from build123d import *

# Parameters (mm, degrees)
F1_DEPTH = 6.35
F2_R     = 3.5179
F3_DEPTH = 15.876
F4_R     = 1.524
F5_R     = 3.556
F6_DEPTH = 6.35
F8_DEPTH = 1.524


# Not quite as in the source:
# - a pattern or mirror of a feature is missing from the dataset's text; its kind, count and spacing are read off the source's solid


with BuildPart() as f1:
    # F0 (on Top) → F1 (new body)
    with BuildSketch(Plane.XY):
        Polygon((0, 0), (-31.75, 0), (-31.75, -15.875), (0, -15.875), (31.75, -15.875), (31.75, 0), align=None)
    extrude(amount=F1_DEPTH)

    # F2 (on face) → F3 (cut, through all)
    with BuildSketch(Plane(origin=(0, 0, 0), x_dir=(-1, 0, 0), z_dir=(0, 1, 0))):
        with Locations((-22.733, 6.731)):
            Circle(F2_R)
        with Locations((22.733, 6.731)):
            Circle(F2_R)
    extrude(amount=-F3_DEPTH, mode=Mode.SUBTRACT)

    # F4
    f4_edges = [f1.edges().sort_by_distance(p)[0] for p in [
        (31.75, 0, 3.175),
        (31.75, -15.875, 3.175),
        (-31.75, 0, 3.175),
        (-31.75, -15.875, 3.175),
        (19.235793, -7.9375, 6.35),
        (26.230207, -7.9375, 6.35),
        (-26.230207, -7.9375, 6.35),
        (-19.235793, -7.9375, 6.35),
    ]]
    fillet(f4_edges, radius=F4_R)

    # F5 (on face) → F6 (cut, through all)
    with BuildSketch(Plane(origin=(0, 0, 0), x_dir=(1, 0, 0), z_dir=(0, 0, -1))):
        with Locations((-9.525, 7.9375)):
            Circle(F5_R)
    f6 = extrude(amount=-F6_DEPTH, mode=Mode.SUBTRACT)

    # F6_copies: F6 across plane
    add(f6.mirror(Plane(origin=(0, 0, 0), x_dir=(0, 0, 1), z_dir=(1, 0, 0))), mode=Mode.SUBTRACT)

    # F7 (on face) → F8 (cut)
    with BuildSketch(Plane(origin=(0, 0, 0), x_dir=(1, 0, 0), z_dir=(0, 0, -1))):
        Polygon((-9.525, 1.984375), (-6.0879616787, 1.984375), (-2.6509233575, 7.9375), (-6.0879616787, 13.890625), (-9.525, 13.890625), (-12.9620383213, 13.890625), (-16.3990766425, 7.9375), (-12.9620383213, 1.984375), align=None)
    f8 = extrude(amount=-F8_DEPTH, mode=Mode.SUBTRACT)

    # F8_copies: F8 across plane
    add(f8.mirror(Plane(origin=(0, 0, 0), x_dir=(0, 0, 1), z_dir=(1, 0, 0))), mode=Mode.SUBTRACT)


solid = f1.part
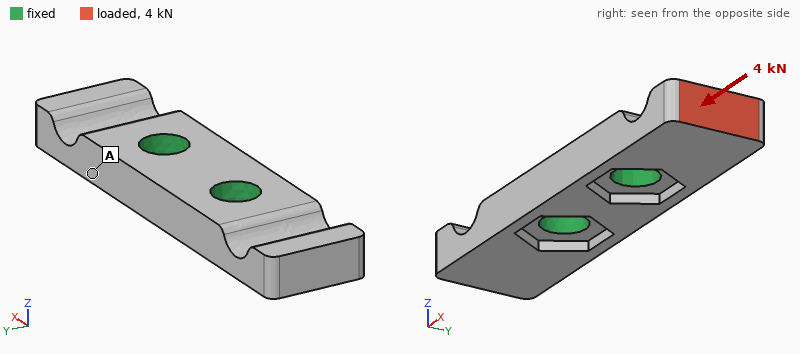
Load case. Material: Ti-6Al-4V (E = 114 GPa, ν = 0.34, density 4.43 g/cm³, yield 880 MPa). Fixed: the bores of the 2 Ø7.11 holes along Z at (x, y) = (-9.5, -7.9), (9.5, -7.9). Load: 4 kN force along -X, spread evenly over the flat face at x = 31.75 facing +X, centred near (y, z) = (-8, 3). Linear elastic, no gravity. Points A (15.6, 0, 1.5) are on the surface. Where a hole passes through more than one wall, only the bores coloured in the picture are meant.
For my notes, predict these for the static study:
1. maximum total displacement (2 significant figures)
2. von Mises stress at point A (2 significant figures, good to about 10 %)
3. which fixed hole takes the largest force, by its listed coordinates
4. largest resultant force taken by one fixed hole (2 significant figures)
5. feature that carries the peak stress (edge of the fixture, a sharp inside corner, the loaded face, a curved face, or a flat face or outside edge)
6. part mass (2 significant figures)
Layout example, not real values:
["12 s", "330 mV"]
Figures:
["59 µm", "42 MPa", "(9.5, -7.9)", "3.7 kN", "a curved face", "23 g"]
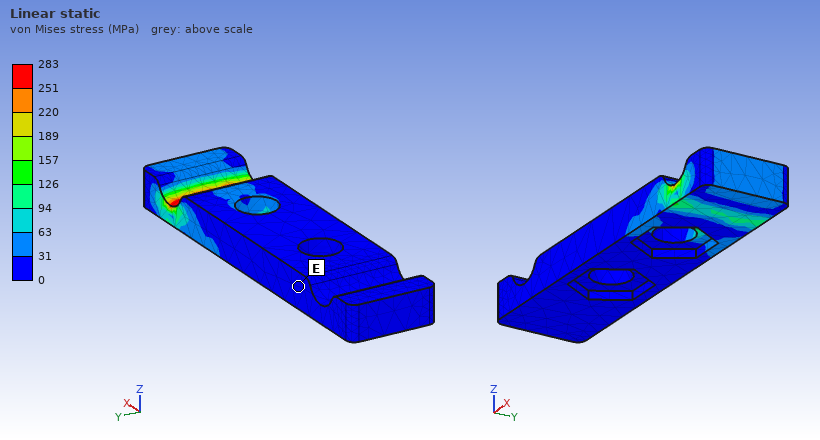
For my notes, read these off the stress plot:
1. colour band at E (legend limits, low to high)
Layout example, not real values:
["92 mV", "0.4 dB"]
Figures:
["0 to 31 MPa"]
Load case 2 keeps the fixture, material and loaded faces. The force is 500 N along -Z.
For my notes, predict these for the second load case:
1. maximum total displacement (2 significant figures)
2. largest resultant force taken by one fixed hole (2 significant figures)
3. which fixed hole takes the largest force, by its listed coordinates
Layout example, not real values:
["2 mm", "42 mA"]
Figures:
["96 µm", "560 N", "(9.5, -7.9)"]
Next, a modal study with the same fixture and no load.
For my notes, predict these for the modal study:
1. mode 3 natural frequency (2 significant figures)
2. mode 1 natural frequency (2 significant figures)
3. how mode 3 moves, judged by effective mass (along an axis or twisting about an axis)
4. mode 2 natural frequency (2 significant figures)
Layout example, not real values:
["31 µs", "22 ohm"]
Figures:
["17 kHz", "8700 Hz", "twisting about Z", "8800 Hz"]
